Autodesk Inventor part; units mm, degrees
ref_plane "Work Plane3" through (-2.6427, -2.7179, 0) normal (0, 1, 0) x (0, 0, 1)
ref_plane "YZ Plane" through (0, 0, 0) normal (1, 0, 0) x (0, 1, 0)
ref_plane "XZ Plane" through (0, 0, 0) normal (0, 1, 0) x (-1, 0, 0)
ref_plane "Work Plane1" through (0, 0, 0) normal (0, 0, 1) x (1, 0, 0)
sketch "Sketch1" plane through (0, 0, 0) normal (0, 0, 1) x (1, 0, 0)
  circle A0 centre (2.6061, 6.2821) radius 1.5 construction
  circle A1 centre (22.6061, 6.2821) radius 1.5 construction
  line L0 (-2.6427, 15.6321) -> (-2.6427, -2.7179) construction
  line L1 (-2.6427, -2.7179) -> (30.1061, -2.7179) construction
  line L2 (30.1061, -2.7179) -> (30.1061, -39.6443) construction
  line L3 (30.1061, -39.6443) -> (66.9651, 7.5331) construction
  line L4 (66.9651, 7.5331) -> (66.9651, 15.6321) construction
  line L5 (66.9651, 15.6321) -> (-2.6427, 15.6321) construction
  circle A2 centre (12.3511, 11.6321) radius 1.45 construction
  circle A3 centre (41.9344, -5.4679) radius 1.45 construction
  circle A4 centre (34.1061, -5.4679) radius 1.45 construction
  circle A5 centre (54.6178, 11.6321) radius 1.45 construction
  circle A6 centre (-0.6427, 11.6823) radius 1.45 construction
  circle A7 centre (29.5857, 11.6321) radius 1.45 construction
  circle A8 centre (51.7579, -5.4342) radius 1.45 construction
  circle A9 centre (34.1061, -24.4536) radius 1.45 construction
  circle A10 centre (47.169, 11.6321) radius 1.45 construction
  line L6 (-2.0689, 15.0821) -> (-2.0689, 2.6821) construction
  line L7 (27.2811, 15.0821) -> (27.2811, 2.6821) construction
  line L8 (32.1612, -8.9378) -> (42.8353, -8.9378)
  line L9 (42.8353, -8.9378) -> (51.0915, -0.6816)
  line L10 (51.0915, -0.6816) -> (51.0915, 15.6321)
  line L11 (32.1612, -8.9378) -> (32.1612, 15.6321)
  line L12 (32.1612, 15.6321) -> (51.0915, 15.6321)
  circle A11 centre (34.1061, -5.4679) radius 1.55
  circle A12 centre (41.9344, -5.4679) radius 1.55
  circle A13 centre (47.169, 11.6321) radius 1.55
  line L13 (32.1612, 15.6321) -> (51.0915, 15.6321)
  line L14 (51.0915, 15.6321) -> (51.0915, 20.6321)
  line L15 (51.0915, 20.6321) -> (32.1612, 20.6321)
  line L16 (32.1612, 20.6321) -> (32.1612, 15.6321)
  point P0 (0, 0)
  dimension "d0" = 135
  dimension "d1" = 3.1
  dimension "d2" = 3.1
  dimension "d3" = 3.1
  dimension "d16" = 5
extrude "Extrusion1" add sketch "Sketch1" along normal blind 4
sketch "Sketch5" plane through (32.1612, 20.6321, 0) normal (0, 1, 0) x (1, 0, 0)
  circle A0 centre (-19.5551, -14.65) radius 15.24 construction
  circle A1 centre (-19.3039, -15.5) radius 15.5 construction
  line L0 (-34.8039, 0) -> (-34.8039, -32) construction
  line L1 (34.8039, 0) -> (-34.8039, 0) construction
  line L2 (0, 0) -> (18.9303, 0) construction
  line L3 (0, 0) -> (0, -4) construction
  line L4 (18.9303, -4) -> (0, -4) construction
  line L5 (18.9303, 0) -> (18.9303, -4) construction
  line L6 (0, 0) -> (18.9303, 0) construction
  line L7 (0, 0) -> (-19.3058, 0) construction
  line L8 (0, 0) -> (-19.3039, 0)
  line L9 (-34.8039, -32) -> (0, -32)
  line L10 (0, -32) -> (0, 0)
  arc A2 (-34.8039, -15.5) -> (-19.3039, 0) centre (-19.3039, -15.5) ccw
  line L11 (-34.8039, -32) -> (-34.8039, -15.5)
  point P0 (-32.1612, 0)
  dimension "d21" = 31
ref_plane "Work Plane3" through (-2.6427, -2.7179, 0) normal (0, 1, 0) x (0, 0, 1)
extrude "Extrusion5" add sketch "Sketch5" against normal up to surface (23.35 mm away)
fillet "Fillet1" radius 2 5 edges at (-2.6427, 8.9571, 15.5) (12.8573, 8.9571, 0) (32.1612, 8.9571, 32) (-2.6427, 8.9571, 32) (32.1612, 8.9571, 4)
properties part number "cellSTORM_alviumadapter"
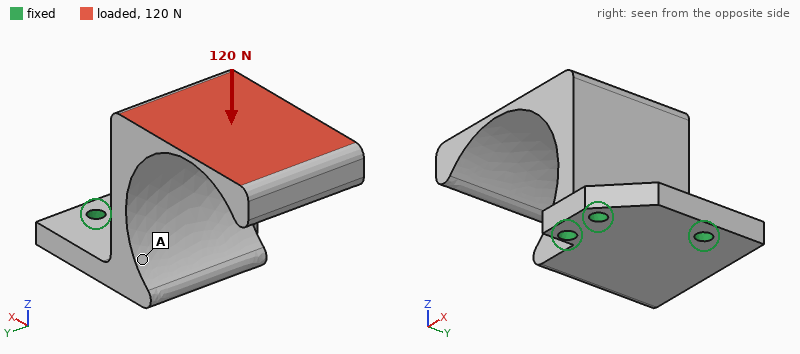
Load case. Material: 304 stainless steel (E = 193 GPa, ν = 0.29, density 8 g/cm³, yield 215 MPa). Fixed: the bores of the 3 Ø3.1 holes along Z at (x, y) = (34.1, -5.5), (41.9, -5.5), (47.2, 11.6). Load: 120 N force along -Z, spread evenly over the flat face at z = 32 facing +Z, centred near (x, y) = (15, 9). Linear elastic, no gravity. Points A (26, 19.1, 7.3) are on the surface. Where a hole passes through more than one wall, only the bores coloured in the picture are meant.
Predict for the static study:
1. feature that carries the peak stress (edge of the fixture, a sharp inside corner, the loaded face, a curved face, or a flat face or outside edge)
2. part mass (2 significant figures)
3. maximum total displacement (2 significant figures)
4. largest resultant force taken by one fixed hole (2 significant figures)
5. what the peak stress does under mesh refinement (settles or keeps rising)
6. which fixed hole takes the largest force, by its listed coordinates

edge of the fixture
70 g
0.18 mm
210 N
keeps rising
(34.1, -5.5)
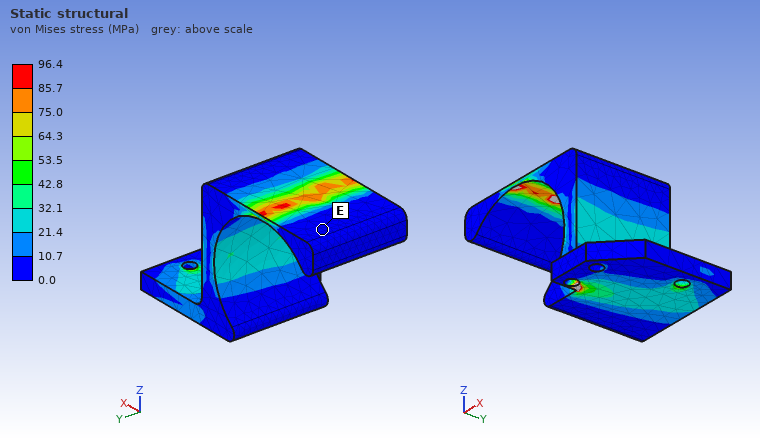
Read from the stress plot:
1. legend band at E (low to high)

0.0 to 10.7 MPa
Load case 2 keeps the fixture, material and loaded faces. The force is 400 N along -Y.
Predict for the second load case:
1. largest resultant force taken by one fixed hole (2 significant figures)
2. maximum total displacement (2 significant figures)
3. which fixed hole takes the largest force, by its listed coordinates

700 N
0.13 mm
(47.2, 11.6)
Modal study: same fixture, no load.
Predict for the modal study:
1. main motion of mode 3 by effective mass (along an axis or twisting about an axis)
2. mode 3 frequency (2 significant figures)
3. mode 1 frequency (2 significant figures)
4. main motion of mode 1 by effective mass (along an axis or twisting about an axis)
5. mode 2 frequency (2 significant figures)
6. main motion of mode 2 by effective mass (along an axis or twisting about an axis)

along Y
2300 Hz
840 Hz
along Z
1500 Hz
along X
